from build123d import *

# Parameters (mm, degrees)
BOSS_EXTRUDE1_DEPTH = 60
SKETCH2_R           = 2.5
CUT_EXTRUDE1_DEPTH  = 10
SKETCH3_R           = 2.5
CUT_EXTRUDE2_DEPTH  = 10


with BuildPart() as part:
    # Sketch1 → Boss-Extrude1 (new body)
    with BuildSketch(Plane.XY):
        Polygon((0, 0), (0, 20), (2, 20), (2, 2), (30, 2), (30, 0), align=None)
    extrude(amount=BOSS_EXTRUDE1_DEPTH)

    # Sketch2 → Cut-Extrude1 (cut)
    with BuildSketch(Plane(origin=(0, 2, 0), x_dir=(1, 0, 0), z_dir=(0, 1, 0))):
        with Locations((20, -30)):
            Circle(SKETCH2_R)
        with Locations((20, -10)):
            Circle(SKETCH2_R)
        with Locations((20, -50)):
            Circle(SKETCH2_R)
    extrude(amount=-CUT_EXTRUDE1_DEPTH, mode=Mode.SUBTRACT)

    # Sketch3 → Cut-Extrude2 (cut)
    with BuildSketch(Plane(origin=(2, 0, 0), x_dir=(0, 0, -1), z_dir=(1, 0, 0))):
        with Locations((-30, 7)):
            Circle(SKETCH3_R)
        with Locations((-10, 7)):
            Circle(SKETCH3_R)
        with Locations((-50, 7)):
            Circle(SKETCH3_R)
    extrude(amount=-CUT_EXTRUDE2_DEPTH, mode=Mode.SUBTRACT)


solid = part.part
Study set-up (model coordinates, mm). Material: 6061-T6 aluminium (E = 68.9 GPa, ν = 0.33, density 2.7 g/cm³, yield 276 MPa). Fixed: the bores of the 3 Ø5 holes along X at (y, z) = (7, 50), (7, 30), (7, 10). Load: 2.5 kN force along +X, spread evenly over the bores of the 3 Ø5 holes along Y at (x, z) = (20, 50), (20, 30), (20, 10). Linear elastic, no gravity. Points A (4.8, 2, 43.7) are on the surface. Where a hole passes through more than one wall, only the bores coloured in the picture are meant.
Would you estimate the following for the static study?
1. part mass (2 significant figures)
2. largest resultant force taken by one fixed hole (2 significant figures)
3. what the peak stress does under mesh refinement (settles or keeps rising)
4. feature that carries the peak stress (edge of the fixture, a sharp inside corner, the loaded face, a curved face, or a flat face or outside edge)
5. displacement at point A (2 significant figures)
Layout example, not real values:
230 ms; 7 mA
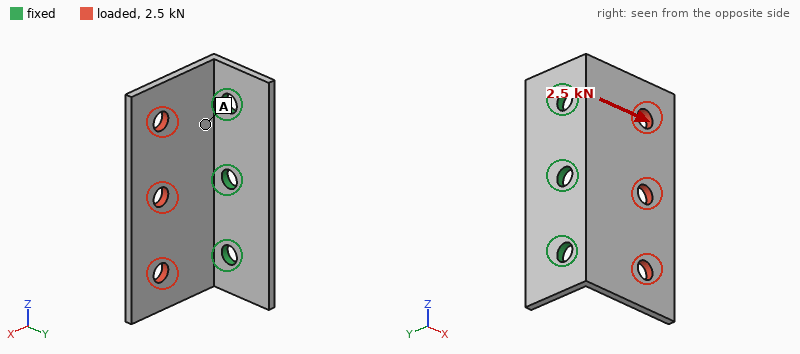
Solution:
15 g; 840 N; keeps rising; edge of the fixture; 0.051 mm
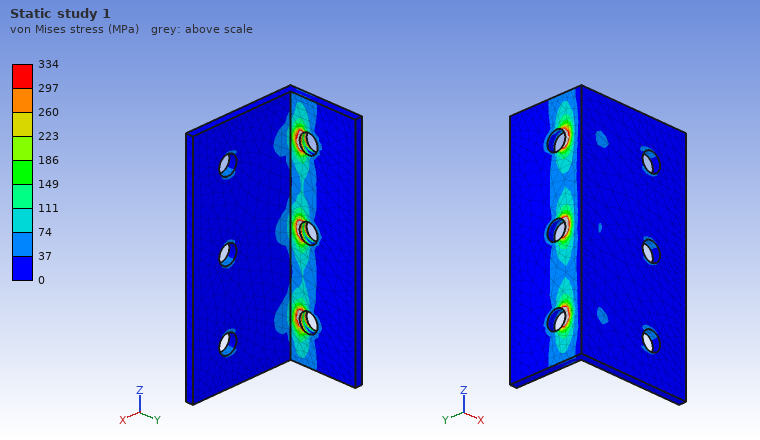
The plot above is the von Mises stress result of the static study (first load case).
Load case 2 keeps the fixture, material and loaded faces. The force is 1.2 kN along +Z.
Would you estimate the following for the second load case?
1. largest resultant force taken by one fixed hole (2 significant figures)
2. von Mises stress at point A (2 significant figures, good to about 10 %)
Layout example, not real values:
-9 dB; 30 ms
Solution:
670 N; 49 MPa
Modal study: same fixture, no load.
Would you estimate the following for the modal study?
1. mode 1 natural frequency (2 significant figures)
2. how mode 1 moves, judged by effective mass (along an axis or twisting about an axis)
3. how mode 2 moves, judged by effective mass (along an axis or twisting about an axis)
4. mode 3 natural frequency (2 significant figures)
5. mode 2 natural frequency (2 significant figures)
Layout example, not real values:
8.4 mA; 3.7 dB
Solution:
1600 Hz; along Y; twisting about X; 5200 Hz; 2600 Hz
